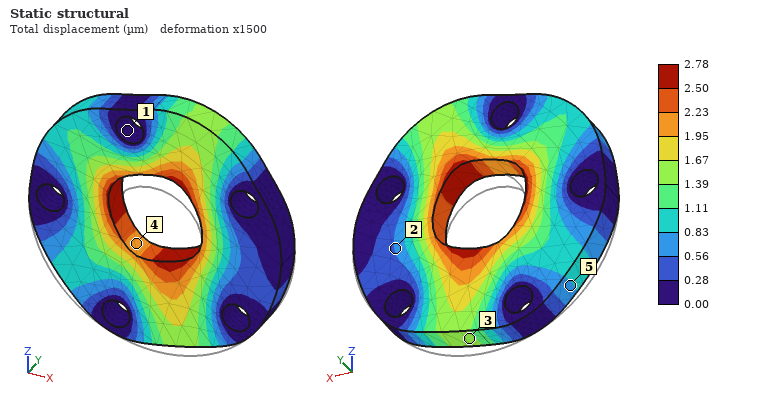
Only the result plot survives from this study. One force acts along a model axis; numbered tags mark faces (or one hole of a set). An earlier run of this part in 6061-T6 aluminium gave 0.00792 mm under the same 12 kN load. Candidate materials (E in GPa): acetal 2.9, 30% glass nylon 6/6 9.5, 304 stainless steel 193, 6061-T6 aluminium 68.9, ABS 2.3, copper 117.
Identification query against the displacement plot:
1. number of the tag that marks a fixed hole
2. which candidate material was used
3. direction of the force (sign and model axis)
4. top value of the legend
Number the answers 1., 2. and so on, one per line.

1. 1
2. 304 stainless steel
3. +Z
4. 2.78 µm
